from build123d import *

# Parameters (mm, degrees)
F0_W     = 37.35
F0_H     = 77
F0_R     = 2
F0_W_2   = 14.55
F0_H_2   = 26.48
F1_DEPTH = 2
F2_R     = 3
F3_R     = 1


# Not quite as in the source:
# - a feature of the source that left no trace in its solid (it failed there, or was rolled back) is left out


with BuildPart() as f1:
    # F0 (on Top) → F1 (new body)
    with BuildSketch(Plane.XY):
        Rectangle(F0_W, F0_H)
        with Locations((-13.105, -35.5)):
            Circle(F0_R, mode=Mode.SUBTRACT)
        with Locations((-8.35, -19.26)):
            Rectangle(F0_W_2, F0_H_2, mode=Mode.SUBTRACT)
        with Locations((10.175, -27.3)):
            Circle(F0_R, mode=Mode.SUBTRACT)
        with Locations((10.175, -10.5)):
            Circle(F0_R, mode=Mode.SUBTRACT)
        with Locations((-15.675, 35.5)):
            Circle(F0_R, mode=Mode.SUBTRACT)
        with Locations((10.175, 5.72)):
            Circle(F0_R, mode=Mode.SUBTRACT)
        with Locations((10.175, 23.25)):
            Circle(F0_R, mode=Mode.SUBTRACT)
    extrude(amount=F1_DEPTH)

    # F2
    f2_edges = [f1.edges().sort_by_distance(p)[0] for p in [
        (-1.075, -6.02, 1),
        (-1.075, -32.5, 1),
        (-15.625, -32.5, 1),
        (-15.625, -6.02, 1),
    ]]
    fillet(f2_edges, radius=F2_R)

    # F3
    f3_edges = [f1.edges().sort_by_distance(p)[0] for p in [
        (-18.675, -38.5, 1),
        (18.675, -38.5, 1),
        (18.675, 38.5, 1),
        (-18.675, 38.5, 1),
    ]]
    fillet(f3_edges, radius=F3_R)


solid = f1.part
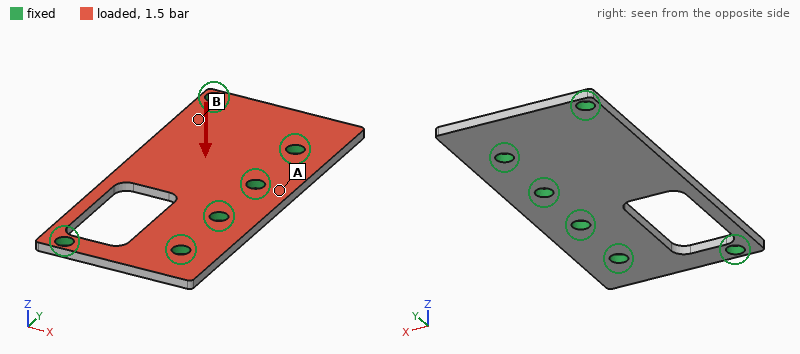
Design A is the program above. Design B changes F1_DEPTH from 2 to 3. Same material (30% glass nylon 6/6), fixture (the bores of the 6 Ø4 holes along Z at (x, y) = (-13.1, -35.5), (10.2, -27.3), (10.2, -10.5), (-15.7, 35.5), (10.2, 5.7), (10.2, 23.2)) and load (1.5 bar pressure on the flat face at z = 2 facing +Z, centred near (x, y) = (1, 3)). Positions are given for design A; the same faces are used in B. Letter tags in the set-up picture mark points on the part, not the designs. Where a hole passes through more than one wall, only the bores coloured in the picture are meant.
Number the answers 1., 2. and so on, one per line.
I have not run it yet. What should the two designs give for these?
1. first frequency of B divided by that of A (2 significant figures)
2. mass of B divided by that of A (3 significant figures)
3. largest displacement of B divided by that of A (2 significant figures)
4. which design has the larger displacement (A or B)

1. 1.5
2. 1.50
3. 0.31
4. A
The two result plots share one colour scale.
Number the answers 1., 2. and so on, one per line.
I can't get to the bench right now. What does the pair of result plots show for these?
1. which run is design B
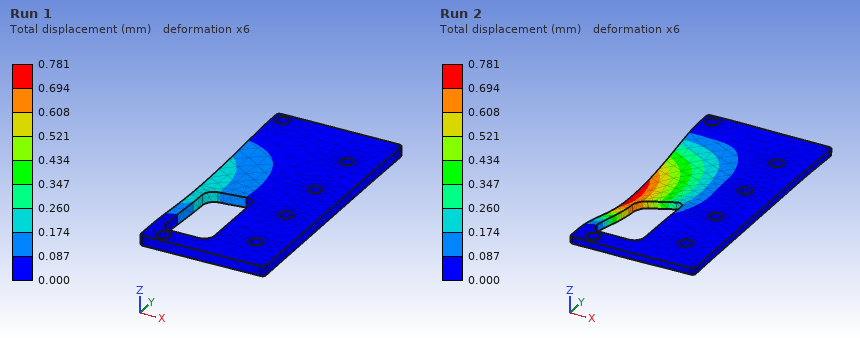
1. Run 1
